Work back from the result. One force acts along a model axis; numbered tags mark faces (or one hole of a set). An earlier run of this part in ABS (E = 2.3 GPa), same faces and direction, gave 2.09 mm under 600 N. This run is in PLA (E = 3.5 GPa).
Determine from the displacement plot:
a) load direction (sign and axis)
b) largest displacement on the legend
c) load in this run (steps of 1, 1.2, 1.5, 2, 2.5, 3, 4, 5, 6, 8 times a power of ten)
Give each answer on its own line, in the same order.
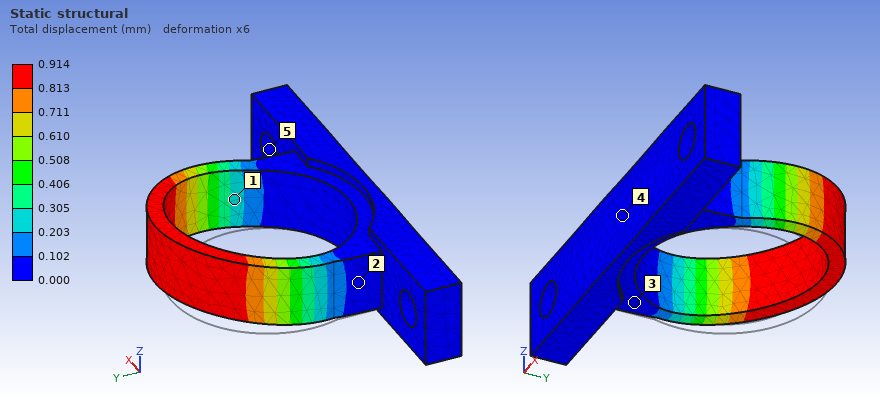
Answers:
+X
0.914 mm
400 N
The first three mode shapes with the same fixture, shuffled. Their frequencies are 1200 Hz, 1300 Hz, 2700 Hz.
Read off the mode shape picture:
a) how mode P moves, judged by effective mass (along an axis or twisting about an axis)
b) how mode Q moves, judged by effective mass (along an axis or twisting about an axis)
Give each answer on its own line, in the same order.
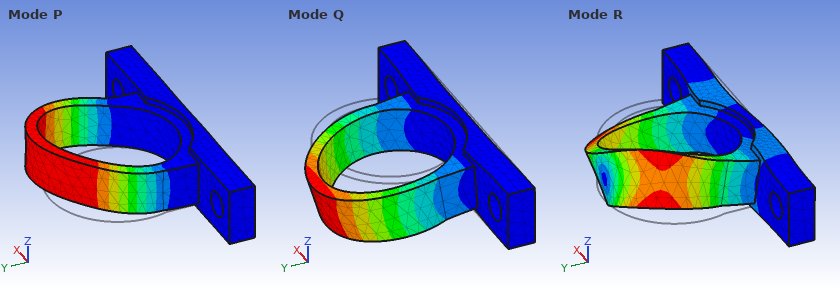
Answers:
along X
along Z
